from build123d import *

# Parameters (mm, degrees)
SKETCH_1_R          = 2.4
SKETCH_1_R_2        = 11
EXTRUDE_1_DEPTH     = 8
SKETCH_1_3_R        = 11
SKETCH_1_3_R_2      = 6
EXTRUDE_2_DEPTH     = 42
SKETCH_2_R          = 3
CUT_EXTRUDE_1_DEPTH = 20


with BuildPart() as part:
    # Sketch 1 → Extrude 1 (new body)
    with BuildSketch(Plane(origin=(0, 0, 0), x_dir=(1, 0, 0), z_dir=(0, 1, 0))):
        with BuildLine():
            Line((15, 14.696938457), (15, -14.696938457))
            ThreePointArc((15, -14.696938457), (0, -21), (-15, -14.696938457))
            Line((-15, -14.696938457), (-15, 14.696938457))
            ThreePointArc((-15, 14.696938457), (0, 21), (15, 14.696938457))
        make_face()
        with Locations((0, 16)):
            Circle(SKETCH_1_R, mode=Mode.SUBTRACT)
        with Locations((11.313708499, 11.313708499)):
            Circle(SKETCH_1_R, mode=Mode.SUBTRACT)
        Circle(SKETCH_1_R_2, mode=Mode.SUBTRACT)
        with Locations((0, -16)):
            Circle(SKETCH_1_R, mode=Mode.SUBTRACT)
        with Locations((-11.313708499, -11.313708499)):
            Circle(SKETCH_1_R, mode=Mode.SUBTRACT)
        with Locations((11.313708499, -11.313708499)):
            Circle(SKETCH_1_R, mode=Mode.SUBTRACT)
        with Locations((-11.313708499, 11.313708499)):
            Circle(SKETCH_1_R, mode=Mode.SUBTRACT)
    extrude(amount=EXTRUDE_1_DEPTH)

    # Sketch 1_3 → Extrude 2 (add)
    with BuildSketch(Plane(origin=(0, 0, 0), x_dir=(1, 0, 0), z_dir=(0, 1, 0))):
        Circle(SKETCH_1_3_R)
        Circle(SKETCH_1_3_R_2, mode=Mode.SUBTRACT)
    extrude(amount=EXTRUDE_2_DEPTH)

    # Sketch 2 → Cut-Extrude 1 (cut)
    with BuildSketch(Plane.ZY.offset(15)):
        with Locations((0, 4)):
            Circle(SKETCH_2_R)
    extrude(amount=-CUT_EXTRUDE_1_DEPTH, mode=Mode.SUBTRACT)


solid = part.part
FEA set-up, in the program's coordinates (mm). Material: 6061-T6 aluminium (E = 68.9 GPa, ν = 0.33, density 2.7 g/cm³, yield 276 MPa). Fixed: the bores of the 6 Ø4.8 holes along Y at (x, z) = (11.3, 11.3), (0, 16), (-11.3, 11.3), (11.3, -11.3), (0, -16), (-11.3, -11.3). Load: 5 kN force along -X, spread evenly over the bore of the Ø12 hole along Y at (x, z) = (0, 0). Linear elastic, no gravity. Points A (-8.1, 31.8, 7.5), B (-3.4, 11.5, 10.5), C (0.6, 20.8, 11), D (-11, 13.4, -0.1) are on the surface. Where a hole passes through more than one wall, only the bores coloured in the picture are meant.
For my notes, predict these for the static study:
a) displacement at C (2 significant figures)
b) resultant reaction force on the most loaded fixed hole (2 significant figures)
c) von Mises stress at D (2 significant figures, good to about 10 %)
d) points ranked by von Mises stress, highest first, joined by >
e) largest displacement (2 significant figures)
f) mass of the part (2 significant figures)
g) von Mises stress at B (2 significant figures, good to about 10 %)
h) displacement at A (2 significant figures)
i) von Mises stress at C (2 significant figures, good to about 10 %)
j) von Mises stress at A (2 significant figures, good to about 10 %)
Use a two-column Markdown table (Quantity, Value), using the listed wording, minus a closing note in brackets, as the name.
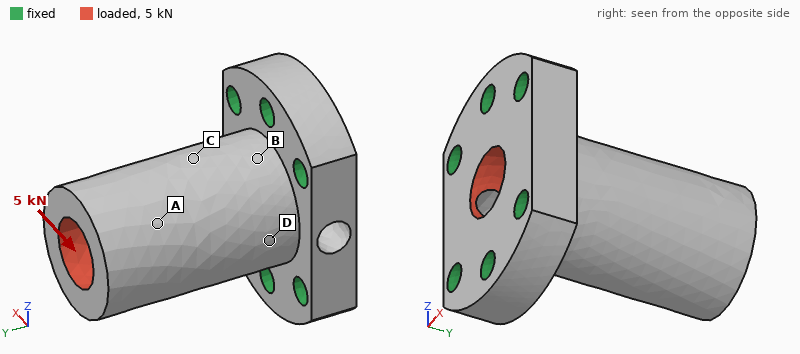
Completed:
| Quantity | Value |
|---|---|
| displacement at C | 29 µm |
| resultant reaction force on the most loaded fixed hole | 2.4 kN |
| von Mises stress at D | 46 MPa |
| points ranked by von Mises stress, highest first, joined by > | D > B > C > A |
| largest displacement | 80 µm |
| mass of the part | 44 g |
| von Mises stress at B | 36 MPa |
| displacement at A | 57 µm |
| von Mises stress at C | 25 MPa |
| von Mises stress at A | 11 MPa |
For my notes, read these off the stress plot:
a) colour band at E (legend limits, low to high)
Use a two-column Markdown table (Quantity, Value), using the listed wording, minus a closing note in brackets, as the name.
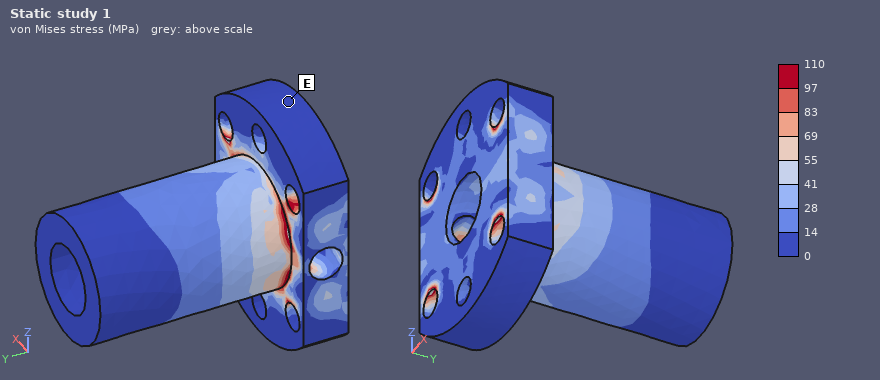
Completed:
| Quantity | Value |
|---|---|
| colour band at E | 0 to 14 MPa |
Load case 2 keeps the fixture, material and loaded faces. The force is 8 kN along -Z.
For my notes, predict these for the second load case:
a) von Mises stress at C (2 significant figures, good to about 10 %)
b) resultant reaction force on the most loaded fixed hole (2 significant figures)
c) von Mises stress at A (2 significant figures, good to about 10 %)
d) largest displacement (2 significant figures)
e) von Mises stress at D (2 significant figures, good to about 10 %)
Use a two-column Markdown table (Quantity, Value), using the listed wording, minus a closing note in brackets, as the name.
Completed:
| Quantity | Value |
|---|---|
| von Mises stress at C | 42 MPa |
| resultant reaction force on the most loaded fixed hole | 3.2 kN |
| von Mises stress at A | 17 MPa |
| largest displacement | 0.11 mm |
| von Mises stress at D | 35 MPa |
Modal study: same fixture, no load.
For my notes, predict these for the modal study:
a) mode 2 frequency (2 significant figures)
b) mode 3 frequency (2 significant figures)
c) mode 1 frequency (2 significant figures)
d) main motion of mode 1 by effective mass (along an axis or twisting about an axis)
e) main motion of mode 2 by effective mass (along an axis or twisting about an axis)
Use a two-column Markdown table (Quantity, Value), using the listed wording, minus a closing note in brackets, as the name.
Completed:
| Quantity | Value |
|---|---|
| mode 2 frequency | 9500 Hz |
| mode 3 frequency | 21 kHz |
| mode 1 frequency | 8700 Hz |
| main motion of mode 1 by effective mass | along X |
| main motion of mode 2 by effective mass | along Z |
